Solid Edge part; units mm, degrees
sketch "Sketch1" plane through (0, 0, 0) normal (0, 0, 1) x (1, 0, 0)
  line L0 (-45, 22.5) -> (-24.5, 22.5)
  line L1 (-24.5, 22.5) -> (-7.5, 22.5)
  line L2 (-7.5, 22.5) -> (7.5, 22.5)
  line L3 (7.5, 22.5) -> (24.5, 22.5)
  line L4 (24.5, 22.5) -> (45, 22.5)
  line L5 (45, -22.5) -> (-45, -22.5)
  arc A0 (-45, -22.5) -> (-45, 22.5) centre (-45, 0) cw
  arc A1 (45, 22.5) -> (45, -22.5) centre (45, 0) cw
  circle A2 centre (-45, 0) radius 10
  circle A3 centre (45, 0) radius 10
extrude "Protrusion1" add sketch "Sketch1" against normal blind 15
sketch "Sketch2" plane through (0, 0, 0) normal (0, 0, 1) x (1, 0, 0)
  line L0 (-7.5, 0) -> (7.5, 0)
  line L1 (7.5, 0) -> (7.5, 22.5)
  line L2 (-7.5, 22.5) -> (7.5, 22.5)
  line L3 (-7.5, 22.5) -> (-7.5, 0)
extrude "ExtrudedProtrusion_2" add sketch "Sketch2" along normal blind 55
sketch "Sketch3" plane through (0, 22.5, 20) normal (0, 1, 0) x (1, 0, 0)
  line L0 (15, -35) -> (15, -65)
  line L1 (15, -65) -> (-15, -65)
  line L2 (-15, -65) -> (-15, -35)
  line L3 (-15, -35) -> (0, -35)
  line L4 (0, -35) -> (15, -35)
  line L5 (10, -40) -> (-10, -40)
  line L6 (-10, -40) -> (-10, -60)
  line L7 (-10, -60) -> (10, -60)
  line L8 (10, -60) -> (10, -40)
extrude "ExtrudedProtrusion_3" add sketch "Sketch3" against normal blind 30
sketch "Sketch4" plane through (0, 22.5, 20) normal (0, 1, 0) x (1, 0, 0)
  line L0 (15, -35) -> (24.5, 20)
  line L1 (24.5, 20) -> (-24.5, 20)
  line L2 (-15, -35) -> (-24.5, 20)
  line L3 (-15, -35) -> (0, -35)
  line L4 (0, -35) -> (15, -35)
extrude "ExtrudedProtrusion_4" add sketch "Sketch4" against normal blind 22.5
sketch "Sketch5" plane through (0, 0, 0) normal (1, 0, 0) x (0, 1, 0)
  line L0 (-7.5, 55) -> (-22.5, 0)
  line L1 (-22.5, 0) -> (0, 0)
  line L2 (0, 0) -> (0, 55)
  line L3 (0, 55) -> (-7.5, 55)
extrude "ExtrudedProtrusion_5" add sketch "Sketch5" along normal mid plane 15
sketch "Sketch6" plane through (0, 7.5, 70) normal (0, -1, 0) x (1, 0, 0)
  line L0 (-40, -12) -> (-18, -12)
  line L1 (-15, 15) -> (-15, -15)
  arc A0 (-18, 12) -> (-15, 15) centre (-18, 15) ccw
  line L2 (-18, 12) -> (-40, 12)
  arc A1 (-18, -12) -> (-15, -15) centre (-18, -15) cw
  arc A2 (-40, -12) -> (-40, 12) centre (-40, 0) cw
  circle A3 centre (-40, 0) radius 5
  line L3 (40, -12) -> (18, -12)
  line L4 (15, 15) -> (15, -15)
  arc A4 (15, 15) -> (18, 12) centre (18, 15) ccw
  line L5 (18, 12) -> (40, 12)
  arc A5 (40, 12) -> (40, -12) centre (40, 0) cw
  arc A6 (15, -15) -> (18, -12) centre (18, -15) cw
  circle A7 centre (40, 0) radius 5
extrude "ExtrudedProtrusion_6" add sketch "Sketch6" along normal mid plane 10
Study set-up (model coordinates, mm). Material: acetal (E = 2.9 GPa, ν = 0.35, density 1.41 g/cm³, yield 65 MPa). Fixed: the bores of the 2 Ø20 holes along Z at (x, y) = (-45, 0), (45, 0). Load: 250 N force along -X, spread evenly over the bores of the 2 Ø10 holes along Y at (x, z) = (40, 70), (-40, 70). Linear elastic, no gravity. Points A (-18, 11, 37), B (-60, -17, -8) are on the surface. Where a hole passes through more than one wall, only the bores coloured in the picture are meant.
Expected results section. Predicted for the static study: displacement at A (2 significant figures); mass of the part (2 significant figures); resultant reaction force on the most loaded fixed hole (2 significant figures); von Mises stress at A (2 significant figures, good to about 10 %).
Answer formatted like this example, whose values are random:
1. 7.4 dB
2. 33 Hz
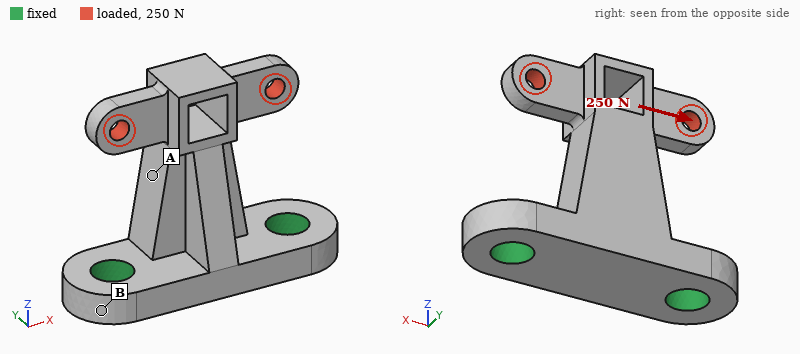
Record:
1. 0.070 mm
2. 230 g
3. 340 N
4. 1.7 MPa
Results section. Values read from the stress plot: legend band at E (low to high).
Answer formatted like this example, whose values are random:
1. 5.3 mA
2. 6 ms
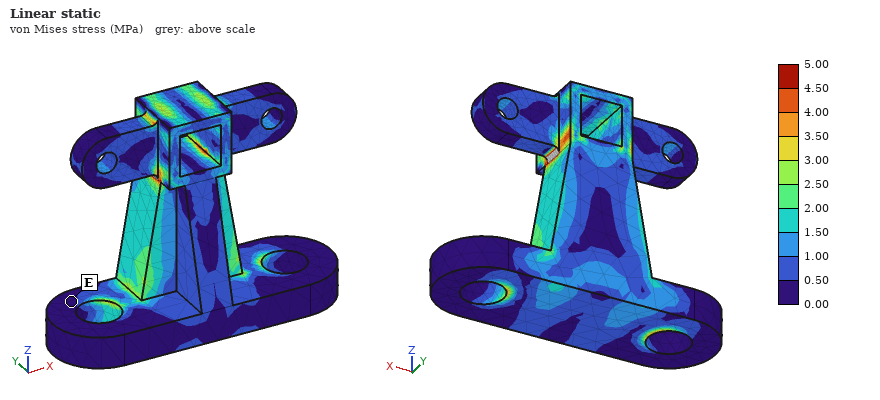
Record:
1. 0.00 to 0.50 MPa
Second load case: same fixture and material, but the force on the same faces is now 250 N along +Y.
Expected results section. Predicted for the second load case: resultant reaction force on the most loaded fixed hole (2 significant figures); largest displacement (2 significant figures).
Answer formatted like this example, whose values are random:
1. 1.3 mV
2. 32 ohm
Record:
1. 130 N
2. 0.80 mm
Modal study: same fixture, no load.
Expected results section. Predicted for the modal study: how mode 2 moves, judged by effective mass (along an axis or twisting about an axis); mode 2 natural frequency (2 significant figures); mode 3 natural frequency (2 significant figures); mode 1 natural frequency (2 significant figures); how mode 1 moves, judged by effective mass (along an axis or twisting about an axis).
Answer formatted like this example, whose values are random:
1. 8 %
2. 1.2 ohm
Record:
1. along X
2. 680 Hz
3. 960 Hz
4. 490 Hz
5. along Y
